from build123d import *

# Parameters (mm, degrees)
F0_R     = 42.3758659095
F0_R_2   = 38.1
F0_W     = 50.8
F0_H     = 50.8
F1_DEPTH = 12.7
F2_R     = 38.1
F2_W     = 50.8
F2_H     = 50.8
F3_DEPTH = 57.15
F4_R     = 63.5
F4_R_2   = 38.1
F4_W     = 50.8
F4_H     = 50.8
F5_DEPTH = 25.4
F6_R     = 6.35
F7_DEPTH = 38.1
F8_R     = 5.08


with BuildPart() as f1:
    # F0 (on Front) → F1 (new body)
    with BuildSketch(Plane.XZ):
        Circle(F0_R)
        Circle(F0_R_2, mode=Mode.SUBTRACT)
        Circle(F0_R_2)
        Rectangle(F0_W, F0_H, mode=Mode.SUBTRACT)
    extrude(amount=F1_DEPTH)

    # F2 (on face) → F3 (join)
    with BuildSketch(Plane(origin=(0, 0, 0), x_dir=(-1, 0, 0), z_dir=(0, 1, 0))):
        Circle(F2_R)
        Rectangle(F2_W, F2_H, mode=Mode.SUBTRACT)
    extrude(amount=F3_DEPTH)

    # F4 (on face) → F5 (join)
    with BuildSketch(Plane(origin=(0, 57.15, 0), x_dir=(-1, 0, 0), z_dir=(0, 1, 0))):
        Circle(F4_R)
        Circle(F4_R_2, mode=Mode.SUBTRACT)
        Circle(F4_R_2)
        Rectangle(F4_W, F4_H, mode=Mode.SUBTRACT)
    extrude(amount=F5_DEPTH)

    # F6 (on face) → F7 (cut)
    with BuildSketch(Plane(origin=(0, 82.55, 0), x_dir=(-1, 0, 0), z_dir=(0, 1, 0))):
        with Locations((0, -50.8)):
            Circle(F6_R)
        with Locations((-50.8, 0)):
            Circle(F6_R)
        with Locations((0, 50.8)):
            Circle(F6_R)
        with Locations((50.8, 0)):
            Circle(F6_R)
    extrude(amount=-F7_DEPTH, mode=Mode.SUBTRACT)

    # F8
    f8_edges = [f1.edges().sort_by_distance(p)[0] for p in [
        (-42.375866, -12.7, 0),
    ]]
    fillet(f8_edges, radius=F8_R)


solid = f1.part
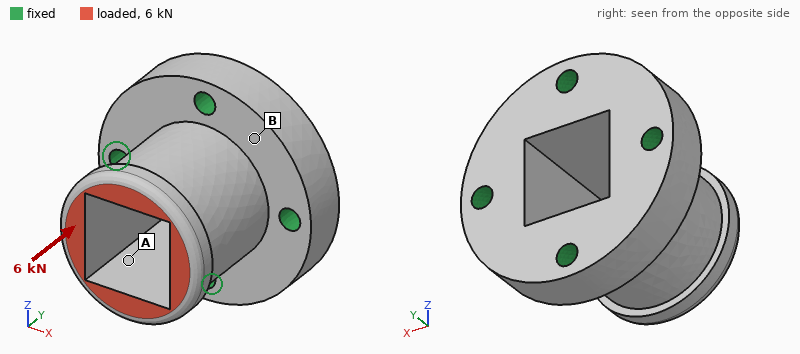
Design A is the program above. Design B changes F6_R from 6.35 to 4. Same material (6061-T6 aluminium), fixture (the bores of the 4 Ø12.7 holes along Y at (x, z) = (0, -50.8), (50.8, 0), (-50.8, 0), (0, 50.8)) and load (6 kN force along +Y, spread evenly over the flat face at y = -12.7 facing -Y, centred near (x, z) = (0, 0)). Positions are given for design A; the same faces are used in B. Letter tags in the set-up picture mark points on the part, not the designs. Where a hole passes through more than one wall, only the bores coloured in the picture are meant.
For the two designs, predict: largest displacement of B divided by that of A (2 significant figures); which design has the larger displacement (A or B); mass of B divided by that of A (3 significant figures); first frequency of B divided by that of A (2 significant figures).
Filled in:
1.1
B
1.02
0.96
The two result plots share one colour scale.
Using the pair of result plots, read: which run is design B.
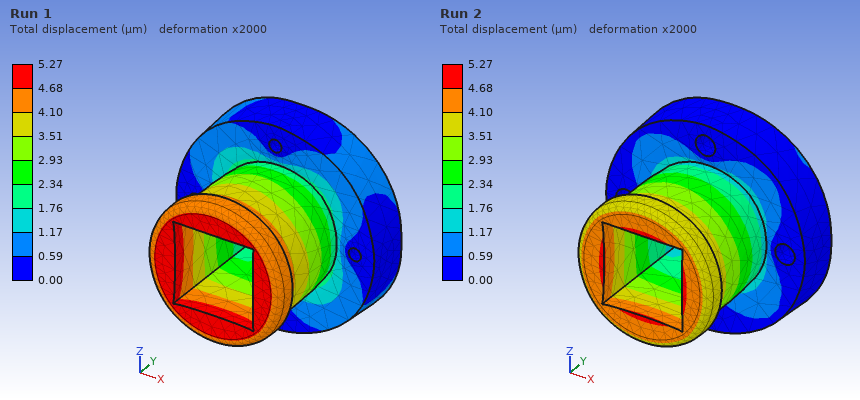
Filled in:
Run 1
